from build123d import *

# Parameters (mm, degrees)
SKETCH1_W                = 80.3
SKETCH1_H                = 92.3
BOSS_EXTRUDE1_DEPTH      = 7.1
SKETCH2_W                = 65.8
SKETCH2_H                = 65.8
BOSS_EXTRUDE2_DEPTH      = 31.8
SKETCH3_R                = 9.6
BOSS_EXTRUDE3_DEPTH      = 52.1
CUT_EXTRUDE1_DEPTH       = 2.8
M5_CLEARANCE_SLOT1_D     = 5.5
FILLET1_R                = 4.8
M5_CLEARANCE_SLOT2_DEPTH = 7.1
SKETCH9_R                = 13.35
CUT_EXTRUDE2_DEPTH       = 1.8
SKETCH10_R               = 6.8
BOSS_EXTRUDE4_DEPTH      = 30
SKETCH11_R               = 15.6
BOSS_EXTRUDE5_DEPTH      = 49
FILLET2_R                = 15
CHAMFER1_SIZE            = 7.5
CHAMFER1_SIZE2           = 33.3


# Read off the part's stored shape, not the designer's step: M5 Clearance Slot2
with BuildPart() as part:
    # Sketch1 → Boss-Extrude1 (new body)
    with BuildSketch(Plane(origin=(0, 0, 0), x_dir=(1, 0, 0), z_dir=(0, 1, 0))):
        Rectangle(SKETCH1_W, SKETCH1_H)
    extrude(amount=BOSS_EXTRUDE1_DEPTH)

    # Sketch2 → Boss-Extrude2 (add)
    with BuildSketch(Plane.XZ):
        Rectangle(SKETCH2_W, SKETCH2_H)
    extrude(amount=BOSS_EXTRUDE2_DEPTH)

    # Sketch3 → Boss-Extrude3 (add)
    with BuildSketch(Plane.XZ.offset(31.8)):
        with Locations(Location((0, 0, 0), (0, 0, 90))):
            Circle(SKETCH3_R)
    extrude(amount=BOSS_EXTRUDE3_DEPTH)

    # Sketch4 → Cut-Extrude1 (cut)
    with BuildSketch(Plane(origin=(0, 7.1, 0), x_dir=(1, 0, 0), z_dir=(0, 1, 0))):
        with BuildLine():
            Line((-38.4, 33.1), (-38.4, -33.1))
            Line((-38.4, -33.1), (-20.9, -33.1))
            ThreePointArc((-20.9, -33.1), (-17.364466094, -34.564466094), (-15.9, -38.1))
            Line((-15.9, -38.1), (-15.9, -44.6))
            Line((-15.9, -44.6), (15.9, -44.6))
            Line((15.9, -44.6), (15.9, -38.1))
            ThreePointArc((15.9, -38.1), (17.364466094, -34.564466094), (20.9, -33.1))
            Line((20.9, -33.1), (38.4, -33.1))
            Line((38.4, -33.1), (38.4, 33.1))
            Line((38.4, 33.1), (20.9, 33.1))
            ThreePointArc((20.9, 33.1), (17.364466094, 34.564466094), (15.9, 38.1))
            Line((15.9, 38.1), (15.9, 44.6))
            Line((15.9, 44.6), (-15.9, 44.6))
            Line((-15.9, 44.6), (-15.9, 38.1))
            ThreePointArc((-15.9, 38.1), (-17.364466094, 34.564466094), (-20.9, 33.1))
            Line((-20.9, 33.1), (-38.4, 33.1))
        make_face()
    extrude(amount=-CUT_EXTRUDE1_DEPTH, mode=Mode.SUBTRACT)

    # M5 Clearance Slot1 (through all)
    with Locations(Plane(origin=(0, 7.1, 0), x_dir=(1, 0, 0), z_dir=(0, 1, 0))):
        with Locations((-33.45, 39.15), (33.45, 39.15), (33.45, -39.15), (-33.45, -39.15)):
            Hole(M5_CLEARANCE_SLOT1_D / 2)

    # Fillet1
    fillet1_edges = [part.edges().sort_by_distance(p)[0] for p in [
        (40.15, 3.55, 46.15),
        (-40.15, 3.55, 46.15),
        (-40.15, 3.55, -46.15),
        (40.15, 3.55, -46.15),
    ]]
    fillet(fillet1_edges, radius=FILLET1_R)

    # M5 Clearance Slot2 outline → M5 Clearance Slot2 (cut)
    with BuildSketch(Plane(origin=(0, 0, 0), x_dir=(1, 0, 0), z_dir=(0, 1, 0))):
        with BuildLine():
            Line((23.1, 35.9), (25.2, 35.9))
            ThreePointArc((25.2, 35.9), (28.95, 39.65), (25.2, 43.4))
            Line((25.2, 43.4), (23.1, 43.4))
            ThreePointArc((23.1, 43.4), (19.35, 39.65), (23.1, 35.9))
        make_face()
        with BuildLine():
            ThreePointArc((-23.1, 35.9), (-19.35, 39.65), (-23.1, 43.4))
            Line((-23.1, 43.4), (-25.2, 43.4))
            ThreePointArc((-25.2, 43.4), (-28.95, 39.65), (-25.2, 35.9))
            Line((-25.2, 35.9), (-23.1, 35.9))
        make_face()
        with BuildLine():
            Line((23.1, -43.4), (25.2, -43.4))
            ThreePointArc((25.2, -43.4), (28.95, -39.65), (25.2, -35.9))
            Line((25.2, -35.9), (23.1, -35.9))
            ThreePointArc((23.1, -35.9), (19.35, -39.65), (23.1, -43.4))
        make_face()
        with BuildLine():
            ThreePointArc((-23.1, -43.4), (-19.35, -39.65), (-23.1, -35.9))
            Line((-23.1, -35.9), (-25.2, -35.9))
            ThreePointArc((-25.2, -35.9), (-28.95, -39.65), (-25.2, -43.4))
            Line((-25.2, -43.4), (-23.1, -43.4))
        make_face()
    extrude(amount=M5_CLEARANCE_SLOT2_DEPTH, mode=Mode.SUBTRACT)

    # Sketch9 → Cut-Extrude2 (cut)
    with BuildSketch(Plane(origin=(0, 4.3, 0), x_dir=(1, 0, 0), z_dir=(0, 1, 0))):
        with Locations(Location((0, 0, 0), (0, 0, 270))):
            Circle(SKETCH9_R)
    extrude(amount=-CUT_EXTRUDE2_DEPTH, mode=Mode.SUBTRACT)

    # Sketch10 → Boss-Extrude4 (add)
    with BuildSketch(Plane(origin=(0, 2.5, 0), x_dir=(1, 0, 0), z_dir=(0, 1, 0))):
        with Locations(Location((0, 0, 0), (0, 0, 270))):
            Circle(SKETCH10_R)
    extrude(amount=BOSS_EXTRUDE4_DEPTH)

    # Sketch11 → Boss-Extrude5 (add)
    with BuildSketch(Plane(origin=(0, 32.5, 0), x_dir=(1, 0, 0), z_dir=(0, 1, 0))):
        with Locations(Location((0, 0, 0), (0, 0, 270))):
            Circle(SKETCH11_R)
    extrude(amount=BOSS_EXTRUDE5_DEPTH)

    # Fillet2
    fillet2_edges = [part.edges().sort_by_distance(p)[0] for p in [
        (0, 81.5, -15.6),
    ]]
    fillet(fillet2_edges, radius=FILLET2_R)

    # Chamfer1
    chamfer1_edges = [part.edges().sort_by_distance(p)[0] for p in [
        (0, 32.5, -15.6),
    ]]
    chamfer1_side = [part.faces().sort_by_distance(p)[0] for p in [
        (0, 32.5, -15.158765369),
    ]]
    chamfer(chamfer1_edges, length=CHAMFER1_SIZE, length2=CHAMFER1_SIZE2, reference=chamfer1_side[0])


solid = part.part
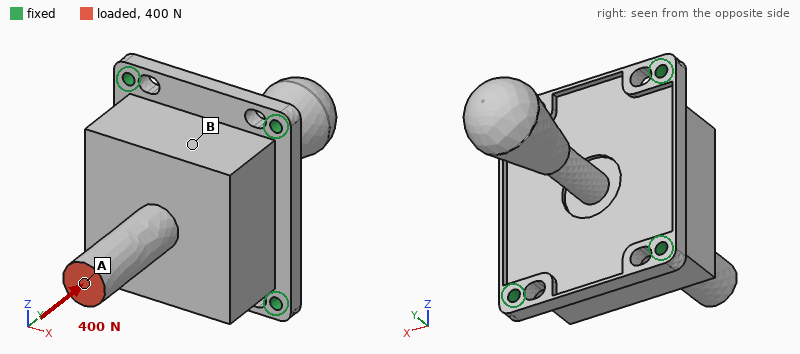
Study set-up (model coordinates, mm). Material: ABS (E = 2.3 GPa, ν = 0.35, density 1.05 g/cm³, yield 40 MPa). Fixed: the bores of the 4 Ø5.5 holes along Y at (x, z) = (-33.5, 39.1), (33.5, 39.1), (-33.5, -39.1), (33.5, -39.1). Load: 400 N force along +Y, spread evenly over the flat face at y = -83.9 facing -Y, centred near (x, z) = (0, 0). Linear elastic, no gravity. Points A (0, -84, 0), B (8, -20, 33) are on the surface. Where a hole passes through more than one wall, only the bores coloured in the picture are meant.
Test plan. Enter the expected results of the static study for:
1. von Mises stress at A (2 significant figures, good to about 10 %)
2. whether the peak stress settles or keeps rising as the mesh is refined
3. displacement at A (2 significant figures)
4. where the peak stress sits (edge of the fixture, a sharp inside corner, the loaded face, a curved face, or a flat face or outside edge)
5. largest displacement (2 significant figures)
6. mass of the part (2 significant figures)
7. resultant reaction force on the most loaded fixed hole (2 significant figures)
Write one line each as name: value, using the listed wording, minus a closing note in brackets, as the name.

von Mises stress at A: 1.4 MPa
whether the peak stress settles or keeps rising as the mesh is refined: keeps rising
displacement at A: 68 µm
where the peak stress sits: edge of the fixture
largest displacement: 68 µm
mass of the part: 220 g
resultant reaction force on the most loaded fixed hole: 120 N
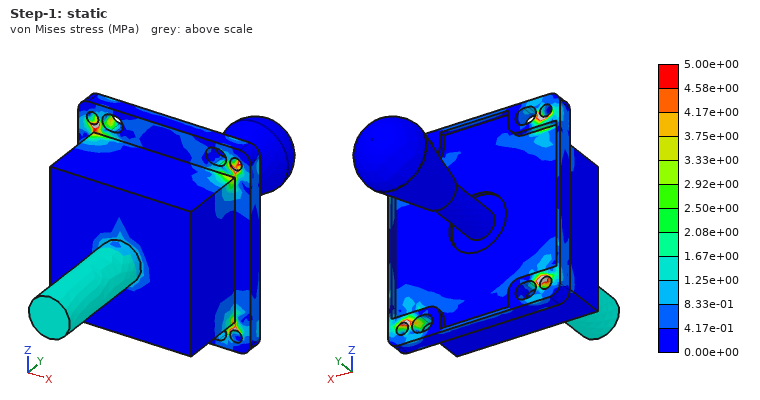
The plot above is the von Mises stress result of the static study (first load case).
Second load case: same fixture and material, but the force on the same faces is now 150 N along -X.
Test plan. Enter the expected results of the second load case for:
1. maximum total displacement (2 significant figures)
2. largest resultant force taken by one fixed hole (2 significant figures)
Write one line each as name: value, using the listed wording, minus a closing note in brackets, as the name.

maximum total displacement: 0.71 mm
largest resultant force taken by one fixed hole: 120 N
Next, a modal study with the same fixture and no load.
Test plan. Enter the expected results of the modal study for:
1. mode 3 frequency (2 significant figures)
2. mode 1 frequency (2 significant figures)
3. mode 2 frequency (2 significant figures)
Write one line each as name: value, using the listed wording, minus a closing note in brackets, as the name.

mode 3 frequency: 950 Hz
mode 1 frequency: 230 Hz
mode 2 frequency: 230 Hz
